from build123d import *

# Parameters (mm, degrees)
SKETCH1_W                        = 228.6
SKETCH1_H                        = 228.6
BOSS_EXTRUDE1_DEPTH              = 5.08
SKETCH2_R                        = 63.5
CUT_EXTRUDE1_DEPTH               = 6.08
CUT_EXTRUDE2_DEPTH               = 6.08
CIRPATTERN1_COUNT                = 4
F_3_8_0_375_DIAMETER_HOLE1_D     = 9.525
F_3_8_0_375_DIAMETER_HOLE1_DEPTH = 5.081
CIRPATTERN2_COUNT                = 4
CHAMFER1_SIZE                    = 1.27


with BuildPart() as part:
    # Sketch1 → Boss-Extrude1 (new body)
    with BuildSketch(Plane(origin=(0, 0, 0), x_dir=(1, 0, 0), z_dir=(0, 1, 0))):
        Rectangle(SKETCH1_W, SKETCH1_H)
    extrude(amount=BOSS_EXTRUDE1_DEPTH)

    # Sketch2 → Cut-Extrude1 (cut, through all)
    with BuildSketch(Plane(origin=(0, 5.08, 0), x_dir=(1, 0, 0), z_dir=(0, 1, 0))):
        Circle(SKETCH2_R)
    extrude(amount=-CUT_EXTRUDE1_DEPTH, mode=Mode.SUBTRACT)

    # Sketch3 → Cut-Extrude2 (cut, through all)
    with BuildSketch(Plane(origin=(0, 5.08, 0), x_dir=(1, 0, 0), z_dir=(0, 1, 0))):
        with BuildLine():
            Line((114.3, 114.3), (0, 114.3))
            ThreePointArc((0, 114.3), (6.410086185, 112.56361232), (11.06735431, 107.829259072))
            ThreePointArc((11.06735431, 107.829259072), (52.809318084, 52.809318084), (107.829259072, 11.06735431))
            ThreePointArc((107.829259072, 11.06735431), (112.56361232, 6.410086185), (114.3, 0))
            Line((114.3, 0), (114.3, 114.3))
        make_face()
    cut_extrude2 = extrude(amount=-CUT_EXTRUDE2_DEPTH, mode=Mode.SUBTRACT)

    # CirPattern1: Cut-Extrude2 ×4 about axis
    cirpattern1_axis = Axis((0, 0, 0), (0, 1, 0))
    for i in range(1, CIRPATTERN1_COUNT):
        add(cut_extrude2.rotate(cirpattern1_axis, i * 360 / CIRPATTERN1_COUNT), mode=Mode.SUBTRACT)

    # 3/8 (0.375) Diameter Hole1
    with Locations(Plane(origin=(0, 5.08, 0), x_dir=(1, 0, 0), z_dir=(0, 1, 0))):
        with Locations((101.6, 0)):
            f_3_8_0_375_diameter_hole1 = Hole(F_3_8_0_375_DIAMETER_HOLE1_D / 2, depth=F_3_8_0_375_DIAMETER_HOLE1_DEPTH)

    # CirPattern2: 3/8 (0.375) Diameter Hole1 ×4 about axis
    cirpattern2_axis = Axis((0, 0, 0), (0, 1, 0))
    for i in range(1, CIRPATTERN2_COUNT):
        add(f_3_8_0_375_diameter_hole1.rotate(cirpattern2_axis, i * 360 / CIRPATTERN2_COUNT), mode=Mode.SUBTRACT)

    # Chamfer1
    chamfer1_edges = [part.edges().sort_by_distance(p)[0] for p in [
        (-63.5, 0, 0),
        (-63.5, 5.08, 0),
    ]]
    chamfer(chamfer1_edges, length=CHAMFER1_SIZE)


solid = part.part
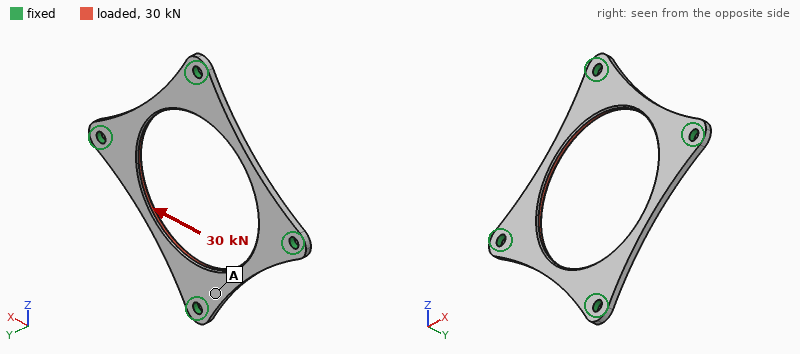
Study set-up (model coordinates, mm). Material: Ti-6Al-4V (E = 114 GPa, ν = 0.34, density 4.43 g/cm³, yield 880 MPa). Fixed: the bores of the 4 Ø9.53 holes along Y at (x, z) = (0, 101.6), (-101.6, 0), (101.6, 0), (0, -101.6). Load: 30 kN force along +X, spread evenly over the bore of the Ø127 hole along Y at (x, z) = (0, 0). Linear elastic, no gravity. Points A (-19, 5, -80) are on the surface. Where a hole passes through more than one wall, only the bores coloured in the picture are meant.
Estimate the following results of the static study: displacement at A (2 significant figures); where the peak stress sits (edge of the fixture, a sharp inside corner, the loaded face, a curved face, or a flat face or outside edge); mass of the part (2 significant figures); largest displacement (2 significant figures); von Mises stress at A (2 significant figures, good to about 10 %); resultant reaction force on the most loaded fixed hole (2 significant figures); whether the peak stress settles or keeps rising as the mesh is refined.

0.086 mm
edge of the fixture
260 g
0.16 mm
36 MPa
9.0 kN
keeps rising
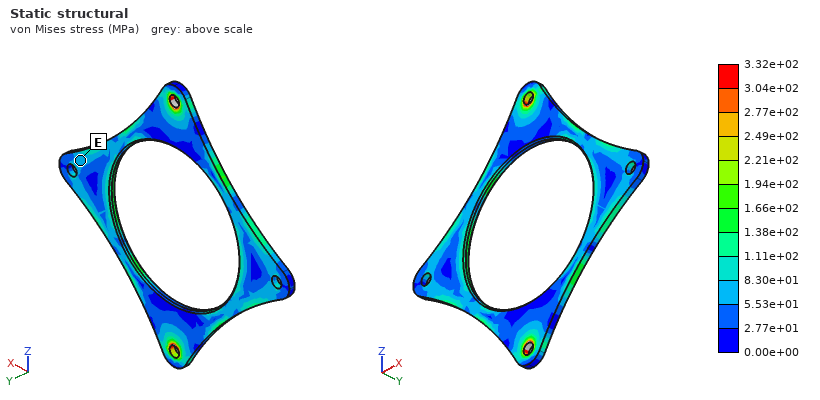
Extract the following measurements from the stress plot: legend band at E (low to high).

5.53e+01 to 8.30e+01 MPa
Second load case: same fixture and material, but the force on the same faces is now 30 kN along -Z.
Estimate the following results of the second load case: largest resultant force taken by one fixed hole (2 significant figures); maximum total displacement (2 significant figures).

9.0 kN
0.16 mm
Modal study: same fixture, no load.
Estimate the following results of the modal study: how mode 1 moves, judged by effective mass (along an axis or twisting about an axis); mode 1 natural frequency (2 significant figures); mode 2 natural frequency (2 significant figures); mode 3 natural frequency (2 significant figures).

along Y
1700 Hz
1700 Hz
1700 Hz
